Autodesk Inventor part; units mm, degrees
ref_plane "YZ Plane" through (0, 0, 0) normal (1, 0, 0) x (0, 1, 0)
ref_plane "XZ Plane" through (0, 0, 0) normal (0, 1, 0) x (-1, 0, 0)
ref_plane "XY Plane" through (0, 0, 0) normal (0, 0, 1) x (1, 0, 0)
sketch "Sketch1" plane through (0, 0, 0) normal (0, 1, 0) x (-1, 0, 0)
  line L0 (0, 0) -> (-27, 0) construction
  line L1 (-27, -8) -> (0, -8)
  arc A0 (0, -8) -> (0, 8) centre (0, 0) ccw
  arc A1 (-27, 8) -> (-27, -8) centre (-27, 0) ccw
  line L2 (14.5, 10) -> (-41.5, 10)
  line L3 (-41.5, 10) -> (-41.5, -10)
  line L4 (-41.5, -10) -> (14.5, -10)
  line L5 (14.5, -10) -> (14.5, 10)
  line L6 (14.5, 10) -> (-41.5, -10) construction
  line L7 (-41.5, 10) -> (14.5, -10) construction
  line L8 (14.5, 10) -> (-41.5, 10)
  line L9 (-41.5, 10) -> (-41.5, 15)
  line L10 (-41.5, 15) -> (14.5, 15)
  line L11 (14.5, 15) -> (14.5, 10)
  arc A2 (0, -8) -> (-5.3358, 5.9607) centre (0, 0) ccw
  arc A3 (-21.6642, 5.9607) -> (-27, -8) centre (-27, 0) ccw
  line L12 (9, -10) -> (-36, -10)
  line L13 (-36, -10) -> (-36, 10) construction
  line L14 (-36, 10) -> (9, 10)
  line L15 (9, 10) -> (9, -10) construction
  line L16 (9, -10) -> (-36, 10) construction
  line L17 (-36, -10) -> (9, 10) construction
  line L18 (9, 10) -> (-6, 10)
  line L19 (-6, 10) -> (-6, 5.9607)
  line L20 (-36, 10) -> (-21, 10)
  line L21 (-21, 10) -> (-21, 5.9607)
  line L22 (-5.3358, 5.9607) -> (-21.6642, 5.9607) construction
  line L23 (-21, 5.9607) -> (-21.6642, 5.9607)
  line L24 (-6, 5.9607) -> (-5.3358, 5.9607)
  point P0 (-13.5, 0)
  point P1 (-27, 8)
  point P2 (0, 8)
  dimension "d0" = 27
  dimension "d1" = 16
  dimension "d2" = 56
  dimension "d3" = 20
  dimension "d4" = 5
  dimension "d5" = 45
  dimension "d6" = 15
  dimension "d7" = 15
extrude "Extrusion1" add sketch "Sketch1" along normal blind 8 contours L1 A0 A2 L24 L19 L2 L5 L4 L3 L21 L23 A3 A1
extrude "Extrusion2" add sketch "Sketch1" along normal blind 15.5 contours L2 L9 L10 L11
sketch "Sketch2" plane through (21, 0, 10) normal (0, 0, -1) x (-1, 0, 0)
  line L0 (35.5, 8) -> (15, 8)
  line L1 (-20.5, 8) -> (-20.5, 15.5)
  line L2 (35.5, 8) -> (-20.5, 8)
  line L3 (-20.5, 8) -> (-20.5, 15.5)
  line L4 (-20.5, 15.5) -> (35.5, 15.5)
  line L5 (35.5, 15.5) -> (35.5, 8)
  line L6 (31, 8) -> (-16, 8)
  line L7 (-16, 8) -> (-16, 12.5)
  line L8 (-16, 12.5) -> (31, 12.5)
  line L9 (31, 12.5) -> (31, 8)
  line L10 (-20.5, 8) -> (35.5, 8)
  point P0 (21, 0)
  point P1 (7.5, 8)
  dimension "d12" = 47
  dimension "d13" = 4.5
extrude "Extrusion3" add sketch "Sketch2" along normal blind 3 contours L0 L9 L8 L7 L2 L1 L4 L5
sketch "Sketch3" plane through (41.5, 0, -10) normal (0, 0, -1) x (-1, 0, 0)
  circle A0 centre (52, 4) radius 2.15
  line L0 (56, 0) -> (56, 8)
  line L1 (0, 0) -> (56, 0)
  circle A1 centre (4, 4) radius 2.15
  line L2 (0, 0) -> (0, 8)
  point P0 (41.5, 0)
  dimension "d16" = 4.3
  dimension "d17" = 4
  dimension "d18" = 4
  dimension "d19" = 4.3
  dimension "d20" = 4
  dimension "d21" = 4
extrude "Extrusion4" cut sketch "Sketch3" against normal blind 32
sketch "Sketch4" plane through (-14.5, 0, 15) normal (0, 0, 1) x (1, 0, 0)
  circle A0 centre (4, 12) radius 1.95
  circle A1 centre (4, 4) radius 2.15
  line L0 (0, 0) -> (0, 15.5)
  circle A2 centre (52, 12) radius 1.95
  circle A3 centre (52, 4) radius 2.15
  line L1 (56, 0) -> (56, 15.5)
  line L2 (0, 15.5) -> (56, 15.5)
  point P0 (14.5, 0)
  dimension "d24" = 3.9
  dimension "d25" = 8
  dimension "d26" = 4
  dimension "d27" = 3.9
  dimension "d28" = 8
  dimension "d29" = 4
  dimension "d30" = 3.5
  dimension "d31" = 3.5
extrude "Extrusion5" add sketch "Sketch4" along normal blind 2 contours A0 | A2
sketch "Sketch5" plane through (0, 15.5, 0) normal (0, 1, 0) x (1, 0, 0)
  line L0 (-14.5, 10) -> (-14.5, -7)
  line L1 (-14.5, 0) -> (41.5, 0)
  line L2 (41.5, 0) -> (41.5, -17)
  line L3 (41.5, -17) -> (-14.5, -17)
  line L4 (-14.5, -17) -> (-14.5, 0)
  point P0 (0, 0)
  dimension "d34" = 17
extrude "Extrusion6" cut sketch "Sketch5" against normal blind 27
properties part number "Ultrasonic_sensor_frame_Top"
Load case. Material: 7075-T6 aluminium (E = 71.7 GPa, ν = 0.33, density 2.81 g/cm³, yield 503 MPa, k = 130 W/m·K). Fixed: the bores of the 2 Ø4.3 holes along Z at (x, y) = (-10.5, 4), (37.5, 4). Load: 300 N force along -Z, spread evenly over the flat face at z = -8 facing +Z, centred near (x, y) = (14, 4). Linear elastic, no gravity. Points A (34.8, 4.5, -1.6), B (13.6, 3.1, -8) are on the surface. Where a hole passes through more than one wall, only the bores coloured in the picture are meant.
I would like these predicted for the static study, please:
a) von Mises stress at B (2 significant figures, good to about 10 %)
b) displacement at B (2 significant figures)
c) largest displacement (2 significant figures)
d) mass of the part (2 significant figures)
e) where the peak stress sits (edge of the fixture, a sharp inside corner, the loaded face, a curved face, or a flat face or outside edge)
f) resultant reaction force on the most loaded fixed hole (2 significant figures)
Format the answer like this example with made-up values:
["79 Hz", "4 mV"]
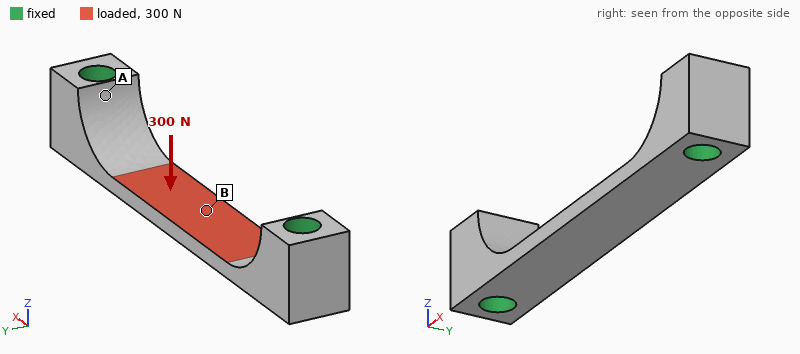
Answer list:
["87 MPa", "0.11 mm", "0.11 mm", "4.7 g", "a curved face", "210 N"]
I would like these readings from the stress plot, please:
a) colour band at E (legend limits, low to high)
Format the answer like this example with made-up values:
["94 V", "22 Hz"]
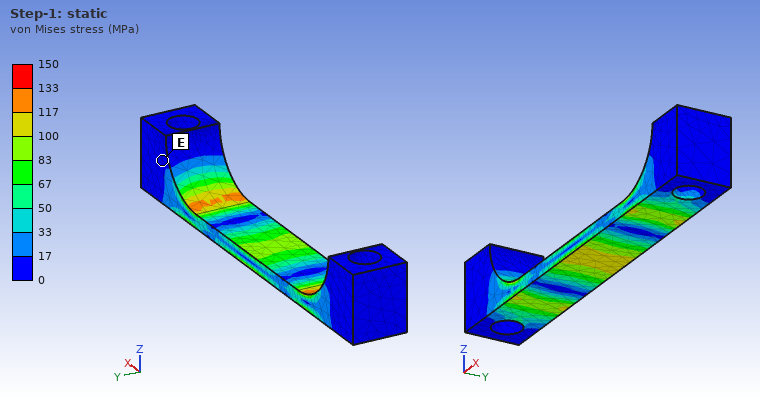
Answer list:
["0 to 17 MPa"]
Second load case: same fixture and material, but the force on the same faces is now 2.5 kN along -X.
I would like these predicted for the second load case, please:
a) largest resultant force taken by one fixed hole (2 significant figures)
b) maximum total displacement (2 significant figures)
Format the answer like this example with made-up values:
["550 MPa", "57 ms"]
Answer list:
["1.3 kN", "23 µm"]
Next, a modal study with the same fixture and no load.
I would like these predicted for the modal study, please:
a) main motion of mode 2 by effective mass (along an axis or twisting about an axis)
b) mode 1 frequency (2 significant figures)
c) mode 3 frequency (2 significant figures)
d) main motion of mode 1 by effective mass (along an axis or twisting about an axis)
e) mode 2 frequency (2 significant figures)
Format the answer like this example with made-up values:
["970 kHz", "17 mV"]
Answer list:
["along Y", "8500 Hz", "21 kHz", "along Z", "19 kHz"]
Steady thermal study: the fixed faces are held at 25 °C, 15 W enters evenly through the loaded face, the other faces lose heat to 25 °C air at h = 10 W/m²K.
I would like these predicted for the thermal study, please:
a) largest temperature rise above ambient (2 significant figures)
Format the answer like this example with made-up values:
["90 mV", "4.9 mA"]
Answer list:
["46 K"]
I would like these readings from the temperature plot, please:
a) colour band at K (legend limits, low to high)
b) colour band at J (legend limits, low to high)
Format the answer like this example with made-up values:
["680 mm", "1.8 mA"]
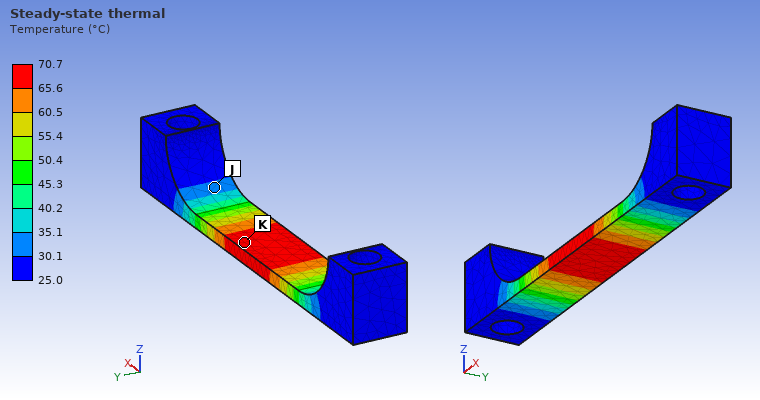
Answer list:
["65.6 to 70.7 °C", "30.1 to 35.1 °C"]
